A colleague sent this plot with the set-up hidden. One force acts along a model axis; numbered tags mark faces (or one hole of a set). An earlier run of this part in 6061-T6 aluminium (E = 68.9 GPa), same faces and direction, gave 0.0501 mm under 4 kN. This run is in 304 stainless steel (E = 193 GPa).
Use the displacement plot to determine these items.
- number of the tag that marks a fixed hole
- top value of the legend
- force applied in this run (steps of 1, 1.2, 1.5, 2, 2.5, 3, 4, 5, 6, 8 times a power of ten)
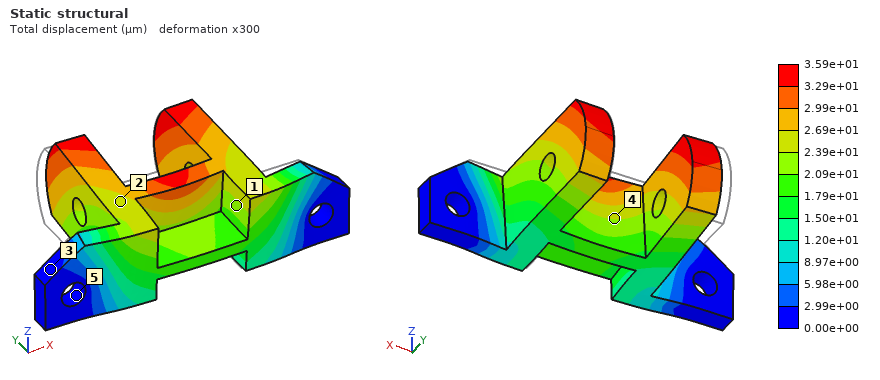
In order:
5
3.59e+01 µm
8 kN
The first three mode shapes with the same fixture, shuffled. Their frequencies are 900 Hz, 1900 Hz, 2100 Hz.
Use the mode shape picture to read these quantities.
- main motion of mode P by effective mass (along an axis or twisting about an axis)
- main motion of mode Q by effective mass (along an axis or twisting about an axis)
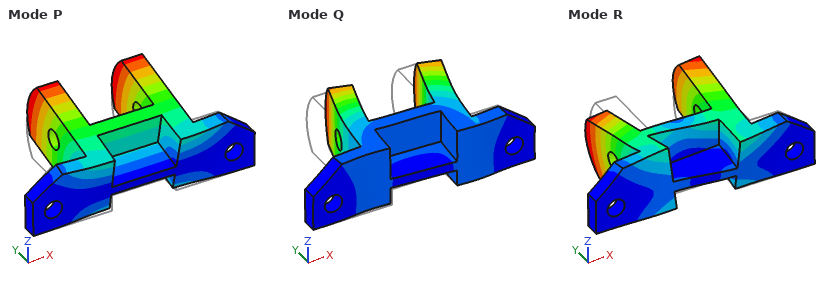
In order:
along Z
along X
